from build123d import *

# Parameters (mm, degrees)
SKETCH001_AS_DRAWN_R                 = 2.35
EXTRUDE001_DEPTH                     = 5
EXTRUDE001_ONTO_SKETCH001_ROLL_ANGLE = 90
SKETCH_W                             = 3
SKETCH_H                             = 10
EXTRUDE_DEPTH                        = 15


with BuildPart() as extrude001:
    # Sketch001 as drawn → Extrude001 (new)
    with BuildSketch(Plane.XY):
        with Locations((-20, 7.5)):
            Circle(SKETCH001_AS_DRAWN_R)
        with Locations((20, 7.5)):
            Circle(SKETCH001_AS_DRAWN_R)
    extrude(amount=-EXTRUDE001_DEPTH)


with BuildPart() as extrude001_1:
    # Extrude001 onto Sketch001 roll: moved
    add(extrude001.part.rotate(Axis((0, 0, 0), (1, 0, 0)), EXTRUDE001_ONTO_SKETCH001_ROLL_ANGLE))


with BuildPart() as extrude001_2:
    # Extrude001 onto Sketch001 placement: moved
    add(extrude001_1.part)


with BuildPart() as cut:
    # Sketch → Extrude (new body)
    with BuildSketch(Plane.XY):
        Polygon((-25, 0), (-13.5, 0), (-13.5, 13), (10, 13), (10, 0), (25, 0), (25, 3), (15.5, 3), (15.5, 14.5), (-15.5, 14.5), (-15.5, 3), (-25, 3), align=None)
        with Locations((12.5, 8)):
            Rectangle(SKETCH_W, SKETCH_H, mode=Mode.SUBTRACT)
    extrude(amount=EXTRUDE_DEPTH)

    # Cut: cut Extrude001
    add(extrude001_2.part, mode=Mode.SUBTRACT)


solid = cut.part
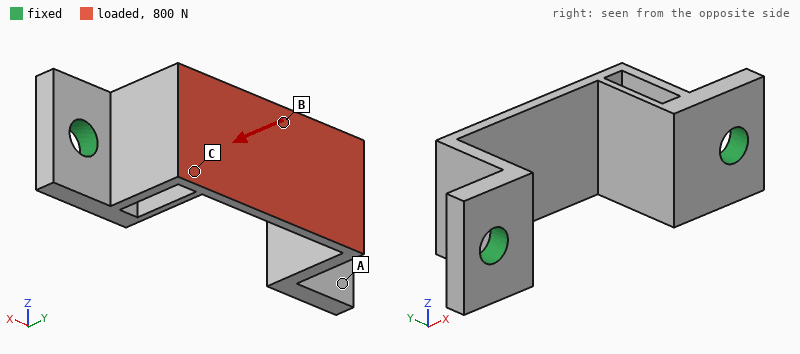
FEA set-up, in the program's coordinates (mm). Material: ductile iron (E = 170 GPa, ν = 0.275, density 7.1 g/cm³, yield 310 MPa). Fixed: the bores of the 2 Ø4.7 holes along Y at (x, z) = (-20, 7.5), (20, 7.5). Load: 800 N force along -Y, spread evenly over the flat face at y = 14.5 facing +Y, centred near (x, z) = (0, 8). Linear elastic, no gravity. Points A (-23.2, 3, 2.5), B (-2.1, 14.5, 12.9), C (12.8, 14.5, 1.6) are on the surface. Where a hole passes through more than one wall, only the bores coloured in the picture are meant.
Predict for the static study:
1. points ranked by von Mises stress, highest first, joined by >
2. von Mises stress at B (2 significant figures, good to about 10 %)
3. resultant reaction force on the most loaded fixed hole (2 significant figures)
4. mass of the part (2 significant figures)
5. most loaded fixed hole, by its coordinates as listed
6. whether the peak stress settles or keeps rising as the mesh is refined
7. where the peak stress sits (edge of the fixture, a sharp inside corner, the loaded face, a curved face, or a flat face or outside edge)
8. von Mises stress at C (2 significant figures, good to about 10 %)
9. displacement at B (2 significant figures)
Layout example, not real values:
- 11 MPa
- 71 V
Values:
- B > C > A
- 150 MPa
- 470 N
- 17 g
- (20, 7.5)
- keeps rising
- edge of the fixture
- 81 MPa
- 58 µm
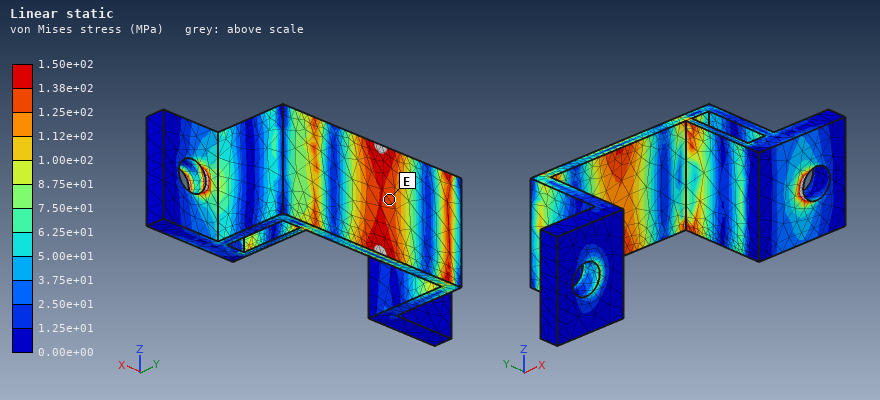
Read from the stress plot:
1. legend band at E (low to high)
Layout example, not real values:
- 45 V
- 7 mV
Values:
- 1.25e+02 to 1.38e+02 MPa
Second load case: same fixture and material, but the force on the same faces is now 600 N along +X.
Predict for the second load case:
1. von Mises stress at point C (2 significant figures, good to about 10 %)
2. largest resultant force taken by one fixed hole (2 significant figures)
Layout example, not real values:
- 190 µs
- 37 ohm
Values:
- 97 MPa
- 320 N
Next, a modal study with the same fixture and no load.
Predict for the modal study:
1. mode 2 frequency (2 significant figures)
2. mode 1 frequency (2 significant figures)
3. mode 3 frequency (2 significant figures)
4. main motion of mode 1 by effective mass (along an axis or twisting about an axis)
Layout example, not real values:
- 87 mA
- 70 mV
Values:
- 9200 Hz
- 5800 Hz
- 9500 Hz
- along X
